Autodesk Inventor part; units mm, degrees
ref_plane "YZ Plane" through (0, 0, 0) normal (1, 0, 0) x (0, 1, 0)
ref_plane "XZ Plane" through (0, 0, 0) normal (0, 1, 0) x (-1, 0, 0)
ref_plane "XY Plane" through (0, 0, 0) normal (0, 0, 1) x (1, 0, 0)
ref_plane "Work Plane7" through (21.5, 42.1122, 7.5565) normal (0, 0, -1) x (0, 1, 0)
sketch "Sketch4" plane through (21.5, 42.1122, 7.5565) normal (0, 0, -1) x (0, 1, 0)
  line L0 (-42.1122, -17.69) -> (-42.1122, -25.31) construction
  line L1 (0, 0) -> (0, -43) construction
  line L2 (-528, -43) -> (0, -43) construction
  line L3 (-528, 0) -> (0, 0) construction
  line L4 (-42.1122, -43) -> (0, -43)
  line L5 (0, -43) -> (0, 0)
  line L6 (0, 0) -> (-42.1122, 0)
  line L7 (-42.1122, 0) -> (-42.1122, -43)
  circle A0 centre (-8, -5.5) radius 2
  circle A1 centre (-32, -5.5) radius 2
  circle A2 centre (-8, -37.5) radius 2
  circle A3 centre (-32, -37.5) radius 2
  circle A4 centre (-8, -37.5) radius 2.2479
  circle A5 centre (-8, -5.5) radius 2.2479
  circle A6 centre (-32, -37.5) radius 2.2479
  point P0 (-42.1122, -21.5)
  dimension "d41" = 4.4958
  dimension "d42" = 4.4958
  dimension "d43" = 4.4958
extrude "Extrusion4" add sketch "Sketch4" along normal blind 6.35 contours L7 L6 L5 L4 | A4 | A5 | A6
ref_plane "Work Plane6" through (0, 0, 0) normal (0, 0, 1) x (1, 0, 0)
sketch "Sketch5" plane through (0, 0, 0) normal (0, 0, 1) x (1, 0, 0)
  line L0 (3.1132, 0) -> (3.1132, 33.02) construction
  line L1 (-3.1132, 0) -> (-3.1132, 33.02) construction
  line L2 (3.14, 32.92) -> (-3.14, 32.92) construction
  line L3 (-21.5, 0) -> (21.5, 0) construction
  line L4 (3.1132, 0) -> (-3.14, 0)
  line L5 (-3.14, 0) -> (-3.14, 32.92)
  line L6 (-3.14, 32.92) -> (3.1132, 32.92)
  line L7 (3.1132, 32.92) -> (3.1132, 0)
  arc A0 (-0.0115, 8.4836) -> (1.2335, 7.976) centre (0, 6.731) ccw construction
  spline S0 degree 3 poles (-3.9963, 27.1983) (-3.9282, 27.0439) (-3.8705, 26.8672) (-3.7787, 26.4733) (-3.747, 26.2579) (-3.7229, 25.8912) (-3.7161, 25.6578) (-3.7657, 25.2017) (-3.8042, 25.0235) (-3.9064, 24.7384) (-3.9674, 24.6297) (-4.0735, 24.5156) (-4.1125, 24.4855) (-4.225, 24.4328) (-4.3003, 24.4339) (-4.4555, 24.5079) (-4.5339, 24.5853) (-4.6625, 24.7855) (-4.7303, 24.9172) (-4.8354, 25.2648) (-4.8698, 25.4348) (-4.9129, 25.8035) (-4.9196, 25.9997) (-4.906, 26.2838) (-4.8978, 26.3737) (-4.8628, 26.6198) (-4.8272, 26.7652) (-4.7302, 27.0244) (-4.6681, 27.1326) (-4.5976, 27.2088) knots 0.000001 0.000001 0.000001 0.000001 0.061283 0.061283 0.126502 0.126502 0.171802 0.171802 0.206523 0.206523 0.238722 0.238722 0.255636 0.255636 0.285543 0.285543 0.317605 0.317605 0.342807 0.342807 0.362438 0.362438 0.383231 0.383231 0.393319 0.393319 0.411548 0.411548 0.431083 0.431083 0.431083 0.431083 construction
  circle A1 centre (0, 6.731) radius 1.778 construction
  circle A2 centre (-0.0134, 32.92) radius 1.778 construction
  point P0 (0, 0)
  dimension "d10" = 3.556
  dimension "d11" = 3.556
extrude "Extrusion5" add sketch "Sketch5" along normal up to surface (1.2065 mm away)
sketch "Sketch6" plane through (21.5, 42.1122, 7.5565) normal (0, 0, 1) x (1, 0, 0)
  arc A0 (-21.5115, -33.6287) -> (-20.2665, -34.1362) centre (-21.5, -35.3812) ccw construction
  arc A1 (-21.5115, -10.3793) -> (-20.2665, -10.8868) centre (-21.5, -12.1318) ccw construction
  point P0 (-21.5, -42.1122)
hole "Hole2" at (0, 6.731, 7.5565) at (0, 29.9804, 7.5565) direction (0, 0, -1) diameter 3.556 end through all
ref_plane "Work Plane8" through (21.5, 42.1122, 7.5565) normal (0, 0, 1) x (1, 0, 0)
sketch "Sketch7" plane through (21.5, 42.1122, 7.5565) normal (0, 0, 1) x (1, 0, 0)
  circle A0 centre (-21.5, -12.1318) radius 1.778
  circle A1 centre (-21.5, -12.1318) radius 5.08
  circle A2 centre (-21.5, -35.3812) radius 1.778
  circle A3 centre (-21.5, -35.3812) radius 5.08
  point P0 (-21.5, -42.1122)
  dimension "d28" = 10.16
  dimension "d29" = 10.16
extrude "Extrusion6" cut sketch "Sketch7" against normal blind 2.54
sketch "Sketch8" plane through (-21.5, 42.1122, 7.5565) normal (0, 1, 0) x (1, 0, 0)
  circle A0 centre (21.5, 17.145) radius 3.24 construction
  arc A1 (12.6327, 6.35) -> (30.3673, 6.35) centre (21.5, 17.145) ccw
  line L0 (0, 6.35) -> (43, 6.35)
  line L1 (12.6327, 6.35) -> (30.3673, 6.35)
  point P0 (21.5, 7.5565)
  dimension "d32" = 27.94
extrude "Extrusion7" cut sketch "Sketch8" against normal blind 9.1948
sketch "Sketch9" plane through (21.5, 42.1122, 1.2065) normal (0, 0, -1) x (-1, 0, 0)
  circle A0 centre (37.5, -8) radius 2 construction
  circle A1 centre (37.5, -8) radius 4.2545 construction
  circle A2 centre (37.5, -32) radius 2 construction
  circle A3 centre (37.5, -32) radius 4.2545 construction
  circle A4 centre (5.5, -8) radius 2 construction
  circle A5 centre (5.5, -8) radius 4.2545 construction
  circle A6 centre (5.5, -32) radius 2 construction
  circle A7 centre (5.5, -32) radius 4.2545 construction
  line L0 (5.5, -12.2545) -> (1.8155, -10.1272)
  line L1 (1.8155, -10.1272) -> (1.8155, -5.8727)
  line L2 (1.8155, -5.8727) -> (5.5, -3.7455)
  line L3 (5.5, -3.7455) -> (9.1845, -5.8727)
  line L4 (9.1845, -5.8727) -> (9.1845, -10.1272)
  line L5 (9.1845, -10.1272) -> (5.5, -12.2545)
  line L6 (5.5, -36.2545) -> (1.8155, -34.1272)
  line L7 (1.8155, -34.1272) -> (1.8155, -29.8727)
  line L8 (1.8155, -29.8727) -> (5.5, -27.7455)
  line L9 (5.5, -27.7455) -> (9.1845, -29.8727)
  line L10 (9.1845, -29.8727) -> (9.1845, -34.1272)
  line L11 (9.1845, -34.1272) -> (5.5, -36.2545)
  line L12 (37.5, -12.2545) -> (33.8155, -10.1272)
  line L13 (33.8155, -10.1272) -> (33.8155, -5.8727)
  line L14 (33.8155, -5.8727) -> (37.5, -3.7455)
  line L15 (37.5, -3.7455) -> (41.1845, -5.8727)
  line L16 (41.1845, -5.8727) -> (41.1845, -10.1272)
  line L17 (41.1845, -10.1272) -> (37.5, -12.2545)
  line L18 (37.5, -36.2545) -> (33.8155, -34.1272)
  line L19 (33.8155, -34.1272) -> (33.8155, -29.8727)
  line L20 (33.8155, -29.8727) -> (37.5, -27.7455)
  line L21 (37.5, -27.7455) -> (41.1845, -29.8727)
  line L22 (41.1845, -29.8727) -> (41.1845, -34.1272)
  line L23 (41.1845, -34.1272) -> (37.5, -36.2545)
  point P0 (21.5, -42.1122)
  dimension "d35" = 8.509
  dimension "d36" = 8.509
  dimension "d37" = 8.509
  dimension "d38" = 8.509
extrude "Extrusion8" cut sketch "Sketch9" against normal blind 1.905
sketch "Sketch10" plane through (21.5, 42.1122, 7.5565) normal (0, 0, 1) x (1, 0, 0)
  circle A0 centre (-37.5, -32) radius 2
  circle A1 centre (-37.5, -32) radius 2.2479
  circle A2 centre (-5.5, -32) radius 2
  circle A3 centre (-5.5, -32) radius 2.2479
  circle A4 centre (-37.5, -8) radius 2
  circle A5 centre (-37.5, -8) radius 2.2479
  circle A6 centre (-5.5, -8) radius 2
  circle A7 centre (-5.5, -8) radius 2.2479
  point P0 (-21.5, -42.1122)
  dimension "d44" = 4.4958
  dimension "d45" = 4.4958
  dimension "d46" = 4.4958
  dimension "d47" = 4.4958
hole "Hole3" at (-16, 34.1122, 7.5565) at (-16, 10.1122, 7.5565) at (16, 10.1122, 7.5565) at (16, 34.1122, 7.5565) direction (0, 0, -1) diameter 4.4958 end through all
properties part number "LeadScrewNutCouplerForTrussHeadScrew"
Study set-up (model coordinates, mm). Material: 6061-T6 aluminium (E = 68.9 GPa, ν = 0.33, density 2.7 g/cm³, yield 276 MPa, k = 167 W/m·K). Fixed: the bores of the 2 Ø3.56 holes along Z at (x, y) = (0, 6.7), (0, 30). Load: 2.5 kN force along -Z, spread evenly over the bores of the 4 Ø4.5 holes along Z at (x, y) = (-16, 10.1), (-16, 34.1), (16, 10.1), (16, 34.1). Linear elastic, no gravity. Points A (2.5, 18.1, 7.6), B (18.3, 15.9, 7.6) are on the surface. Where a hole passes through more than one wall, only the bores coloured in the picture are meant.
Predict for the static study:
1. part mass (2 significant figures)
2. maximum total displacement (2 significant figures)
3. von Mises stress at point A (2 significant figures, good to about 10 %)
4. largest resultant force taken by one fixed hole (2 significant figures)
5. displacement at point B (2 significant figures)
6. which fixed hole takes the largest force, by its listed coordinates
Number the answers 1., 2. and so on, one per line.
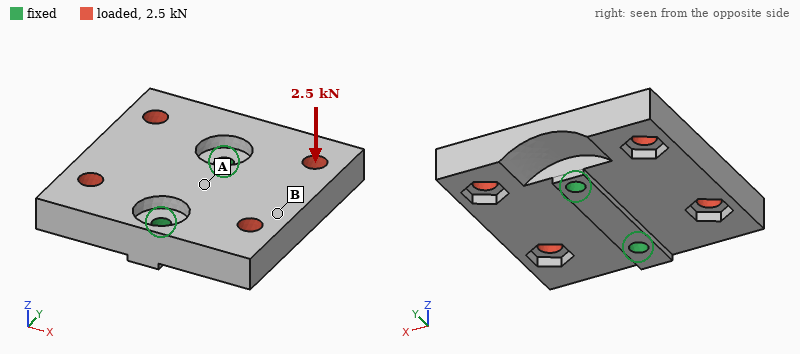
1. 28 g
2. 80 µm
3. 72 MPa
4. 1.6 kN
5. 46 µm
6. (0, 30)
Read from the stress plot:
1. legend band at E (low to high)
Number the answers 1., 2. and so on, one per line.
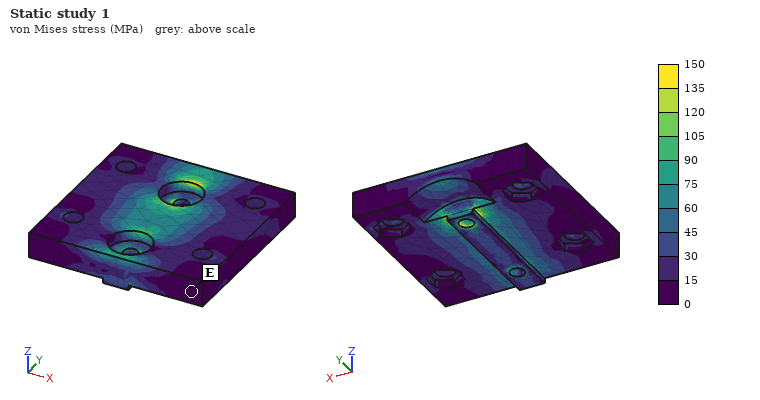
1. 0 to 15 MPa
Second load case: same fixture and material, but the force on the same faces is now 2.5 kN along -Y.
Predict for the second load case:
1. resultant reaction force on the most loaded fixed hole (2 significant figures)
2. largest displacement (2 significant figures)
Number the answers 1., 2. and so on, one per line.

1. 1.3 kN
2. 13 µm
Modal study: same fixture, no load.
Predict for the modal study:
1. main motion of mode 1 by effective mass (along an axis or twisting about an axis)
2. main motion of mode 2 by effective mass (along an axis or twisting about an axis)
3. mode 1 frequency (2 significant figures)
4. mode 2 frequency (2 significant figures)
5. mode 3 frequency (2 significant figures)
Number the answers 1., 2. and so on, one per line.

1. twisting about Y
2. along Z
3. 5800 Hz
4. 9400 Hz
5. 11 kHz
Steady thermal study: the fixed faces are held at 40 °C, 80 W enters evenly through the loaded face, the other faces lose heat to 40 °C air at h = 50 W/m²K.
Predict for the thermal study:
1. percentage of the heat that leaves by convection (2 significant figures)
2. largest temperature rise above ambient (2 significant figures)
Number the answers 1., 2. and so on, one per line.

1. 5.8 %
2. 32 K
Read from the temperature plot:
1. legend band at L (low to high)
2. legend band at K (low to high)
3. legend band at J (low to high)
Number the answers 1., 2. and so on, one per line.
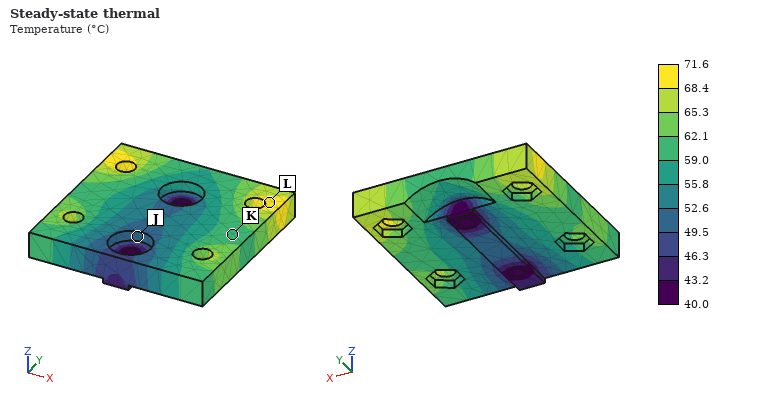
1. 68.4 to 71.6 °C
2. 59.0 to 62.1 °C
3. 49.5 to 52.6 °C
